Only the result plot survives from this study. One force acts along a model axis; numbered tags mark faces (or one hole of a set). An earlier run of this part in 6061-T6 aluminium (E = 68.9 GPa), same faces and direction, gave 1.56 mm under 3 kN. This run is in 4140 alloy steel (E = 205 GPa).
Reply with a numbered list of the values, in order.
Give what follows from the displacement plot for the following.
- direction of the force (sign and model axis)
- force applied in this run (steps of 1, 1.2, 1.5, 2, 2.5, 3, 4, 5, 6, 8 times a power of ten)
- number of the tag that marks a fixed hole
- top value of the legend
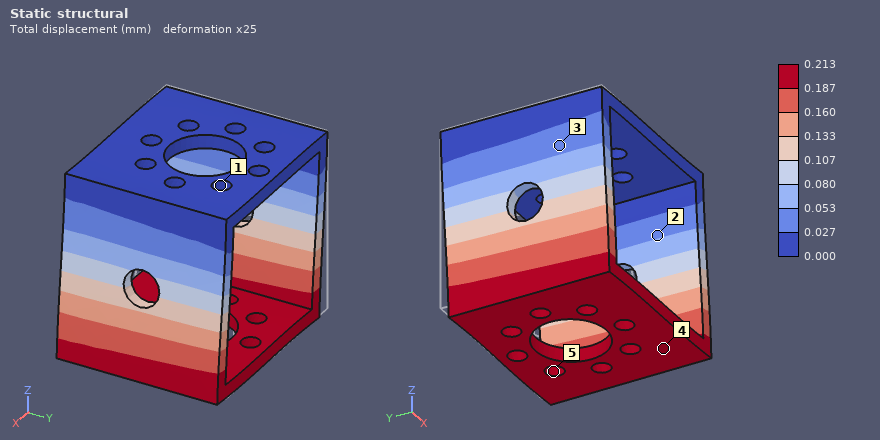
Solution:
1. +X
2. 1.2 kN
3. 1
4. 0.213 mm
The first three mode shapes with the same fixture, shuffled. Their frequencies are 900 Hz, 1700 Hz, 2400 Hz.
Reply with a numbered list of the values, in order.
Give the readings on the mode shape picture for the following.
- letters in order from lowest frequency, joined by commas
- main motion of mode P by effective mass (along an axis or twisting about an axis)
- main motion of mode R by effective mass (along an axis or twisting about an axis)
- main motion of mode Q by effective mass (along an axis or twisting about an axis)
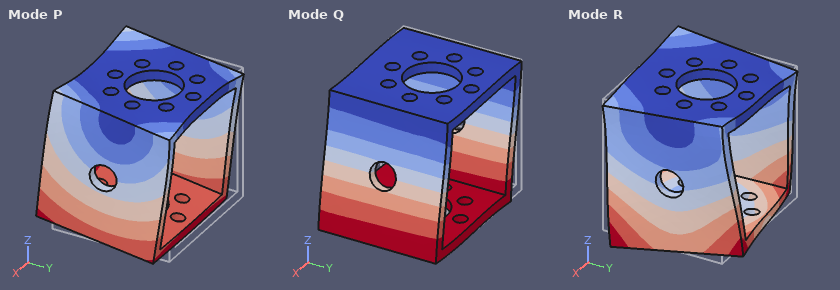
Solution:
1. Q, P, R
2. along Y
3. twisting about Z
4. along X
